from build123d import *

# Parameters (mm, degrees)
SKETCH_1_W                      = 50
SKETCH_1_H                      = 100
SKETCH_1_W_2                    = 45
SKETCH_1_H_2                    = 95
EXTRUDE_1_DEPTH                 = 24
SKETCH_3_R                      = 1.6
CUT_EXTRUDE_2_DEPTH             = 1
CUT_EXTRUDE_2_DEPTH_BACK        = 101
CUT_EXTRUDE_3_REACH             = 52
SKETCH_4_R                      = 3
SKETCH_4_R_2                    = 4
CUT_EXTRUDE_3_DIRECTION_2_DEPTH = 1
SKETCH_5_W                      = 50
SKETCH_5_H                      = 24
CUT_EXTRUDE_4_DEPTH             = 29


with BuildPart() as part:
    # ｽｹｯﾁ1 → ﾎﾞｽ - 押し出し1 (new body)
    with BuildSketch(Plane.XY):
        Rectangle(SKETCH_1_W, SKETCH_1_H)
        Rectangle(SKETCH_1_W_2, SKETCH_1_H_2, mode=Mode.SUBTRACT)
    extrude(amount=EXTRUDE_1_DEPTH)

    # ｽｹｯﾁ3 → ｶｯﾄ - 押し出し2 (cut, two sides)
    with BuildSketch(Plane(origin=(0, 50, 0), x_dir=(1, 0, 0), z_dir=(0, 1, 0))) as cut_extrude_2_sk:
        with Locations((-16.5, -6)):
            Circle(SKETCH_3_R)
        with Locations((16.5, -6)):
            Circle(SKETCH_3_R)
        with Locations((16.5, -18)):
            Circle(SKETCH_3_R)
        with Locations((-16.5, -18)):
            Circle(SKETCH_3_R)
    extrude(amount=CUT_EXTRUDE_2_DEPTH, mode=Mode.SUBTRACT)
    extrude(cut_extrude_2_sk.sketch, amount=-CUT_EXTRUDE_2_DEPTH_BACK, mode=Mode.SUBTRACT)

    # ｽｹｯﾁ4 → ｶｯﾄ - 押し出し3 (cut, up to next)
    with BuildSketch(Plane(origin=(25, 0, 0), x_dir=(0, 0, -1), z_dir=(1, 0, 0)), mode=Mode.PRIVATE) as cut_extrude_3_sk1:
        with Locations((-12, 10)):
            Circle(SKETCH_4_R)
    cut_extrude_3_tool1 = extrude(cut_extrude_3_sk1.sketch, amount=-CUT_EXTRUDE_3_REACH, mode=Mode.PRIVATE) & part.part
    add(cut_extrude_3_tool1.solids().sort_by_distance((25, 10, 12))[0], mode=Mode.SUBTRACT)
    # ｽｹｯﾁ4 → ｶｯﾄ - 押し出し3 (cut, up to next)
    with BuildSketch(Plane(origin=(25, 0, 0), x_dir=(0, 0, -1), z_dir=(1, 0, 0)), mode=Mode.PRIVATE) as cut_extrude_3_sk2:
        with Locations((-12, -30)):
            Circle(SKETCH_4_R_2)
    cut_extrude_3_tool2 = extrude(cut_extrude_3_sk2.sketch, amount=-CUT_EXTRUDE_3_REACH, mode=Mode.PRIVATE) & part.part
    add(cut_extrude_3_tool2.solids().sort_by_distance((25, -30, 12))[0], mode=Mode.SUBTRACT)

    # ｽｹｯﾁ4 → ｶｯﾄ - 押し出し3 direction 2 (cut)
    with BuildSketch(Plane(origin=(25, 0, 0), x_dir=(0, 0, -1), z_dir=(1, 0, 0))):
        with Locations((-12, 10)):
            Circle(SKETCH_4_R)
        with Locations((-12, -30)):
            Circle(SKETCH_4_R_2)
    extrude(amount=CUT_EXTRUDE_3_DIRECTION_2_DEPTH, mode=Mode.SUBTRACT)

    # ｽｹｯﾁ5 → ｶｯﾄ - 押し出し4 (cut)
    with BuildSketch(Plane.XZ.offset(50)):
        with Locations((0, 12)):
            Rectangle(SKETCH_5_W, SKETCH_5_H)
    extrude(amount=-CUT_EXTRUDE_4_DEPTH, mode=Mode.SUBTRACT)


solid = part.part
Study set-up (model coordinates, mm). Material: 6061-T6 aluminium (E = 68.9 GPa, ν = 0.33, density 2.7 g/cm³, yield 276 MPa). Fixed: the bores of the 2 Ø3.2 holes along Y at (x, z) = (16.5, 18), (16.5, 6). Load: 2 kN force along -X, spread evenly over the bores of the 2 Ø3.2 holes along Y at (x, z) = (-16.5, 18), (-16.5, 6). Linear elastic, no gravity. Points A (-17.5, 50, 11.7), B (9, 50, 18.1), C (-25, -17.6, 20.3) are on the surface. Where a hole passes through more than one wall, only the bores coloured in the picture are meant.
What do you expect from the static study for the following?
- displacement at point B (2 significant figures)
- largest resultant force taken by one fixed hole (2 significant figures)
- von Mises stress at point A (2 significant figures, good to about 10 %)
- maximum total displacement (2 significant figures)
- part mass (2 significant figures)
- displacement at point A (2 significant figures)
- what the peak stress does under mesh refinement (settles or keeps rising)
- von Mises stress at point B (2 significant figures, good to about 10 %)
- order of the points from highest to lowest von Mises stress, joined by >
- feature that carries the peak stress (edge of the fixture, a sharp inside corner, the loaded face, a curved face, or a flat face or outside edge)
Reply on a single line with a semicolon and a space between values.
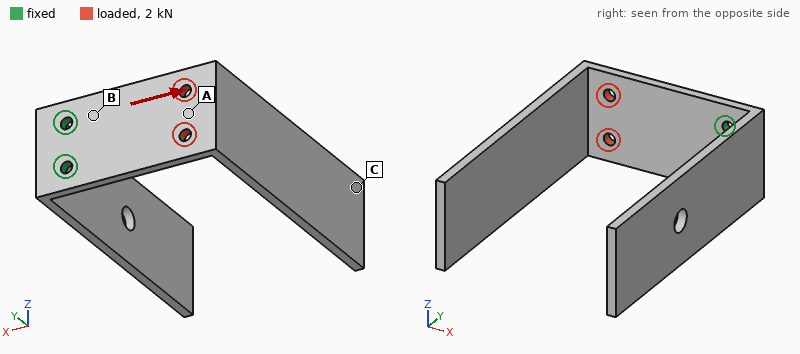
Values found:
4.2 µm; 1.0 kN; 17 MPa; 22 µm; 30 g; 16 µm; keeps rising; 38 MPa; B > A > C; edge of the fixture
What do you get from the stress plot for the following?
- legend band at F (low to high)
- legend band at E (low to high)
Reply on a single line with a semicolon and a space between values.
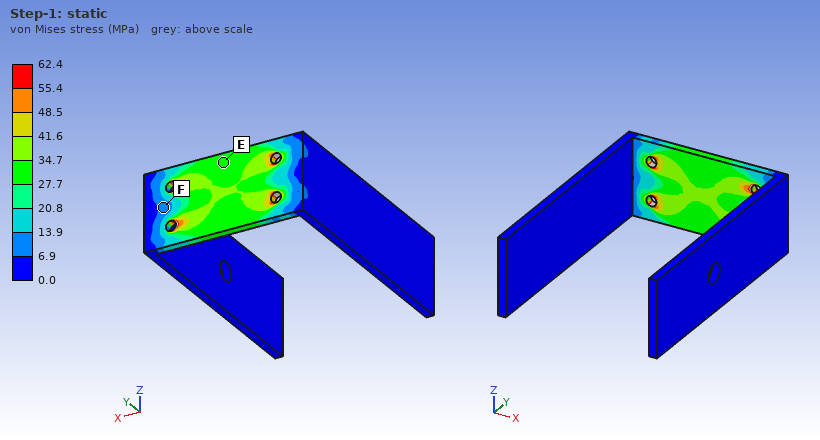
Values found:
6.9 to 13.9 MPa; 27.7 to 34.7 MPa
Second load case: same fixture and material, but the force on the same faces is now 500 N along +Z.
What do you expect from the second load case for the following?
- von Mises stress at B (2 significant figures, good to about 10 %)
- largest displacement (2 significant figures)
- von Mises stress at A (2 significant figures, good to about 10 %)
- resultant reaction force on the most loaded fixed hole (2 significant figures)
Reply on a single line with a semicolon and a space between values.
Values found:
37 MPa; 68 µm; 11 MPa; 1.2 kN
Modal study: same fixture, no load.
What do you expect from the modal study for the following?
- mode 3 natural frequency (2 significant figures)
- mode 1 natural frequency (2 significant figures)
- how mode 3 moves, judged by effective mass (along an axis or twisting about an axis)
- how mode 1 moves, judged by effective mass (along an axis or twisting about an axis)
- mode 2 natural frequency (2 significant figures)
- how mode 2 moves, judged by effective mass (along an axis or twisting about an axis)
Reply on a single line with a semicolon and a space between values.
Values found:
370 Hz; 220 Hz; along X; along X; 350 Hz; along Z
